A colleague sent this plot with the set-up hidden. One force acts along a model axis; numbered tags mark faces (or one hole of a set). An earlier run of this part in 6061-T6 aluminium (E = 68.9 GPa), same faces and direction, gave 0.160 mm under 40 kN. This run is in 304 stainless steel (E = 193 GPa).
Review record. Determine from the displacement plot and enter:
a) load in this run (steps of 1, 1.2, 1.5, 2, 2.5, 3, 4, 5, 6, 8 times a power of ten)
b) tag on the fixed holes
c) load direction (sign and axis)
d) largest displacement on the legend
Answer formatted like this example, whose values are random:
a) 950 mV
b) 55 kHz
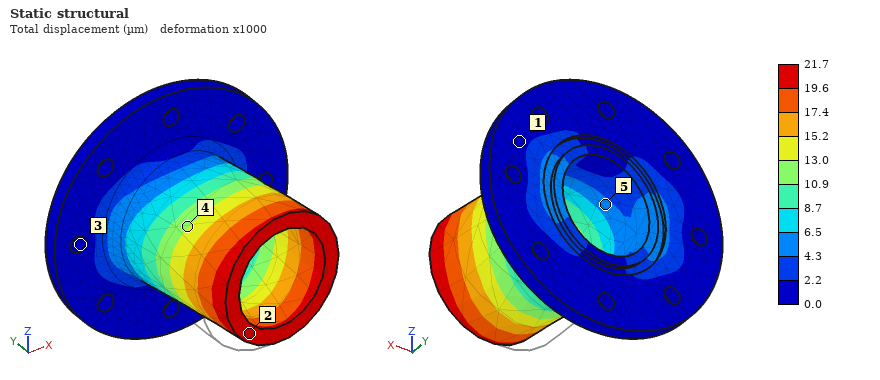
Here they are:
a) 15 kN
b) 3
c) +X
d) 21.7 µm
